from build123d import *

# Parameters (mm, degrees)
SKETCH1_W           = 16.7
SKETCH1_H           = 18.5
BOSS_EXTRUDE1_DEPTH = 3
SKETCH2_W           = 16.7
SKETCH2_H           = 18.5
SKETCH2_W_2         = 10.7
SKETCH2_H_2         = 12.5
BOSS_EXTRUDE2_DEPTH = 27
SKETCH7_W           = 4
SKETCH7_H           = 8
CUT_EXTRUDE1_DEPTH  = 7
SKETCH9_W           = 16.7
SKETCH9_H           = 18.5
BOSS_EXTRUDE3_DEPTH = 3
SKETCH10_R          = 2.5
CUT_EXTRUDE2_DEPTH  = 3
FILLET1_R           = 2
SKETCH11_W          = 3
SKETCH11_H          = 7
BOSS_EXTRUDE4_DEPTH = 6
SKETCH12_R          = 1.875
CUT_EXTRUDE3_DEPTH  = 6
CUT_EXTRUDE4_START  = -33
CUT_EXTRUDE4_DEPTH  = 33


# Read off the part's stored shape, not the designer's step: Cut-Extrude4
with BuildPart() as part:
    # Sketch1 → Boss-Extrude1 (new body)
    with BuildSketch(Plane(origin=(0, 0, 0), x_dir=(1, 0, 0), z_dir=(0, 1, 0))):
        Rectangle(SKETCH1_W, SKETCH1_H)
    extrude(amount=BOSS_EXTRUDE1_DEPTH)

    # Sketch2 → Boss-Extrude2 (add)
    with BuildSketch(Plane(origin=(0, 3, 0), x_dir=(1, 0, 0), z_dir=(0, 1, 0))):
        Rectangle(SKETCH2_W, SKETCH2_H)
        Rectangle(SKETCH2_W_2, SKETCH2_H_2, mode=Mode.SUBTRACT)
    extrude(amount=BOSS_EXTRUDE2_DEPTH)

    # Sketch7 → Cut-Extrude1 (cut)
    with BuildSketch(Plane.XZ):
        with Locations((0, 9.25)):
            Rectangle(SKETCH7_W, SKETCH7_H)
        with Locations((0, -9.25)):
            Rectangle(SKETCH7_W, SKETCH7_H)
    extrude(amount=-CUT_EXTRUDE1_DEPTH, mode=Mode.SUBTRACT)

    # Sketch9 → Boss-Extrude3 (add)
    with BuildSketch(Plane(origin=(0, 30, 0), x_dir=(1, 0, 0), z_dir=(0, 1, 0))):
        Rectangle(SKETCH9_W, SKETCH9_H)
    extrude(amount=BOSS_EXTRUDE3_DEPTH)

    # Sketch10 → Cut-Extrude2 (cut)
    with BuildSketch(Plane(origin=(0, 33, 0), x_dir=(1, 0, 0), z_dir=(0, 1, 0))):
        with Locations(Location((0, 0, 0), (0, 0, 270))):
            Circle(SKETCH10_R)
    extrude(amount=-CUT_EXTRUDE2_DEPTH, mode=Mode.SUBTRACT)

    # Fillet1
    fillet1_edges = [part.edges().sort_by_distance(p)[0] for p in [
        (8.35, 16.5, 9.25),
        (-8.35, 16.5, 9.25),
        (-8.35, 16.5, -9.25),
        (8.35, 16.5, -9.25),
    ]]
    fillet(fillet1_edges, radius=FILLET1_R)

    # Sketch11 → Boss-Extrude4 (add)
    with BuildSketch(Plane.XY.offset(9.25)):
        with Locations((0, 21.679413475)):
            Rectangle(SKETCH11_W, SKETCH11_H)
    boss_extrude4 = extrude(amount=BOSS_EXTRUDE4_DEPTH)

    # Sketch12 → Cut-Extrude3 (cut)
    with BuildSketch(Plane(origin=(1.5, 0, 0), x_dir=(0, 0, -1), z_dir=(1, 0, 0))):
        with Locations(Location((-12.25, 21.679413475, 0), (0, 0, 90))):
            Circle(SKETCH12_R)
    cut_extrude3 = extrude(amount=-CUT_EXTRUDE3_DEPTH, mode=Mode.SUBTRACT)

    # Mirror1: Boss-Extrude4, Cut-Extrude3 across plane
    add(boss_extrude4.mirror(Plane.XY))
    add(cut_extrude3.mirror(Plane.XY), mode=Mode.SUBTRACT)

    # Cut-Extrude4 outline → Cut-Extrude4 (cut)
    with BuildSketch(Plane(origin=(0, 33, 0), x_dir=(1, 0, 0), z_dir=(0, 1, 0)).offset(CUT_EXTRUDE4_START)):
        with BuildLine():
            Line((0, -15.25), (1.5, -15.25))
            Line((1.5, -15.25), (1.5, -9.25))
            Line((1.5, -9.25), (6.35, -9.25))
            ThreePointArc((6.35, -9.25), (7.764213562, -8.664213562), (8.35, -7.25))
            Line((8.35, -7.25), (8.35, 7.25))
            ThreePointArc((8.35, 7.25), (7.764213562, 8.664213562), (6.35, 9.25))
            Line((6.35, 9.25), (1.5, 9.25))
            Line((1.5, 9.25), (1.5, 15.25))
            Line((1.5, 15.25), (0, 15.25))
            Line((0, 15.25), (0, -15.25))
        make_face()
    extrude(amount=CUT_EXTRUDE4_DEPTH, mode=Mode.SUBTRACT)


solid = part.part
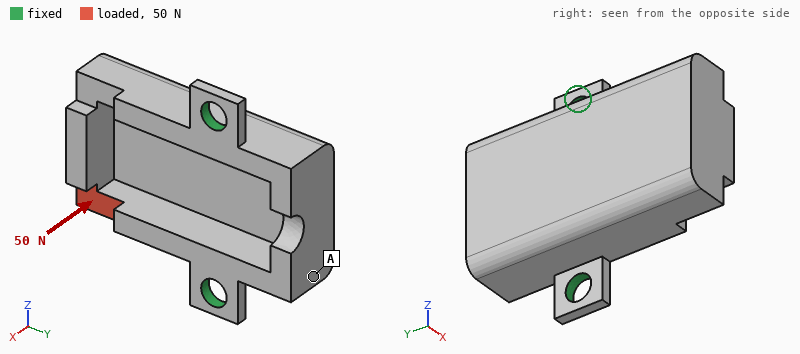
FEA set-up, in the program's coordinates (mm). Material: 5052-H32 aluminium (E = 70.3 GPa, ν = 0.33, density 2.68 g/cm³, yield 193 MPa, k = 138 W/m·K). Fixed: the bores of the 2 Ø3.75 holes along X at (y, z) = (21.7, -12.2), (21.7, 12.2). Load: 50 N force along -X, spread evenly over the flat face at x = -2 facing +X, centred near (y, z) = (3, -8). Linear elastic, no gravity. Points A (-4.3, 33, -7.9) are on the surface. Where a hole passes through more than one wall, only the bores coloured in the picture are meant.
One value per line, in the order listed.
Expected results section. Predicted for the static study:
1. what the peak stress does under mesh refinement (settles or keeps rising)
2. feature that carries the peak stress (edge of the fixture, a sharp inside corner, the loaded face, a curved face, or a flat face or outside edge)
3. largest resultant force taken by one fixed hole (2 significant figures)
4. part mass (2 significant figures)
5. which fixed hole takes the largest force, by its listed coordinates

keeps rising
edge of the fixture
47 N
8.6 g
(21.7, -12.2)
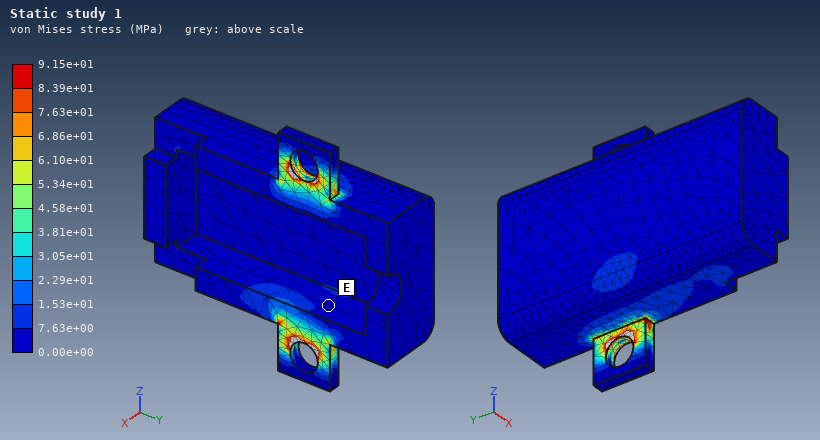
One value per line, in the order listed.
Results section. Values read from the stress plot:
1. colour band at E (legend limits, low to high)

0.00e+00 to 7.63e+00 MPa
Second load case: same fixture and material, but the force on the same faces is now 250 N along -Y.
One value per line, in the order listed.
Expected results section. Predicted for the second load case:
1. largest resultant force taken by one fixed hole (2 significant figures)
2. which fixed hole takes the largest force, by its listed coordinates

220 N
(21.7, -12.2)
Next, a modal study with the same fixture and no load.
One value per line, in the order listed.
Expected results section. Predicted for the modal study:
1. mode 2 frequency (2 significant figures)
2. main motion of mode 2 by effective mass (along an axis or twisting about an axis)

9000 Hz
along Z
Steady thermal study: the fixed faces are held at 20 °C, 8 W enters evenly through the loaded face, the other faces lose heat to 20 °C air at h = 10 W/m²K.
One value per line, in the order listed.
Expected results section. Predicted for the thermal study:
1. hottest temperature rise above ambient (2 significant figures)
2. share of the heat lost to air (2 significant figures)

31 K
3.8 %
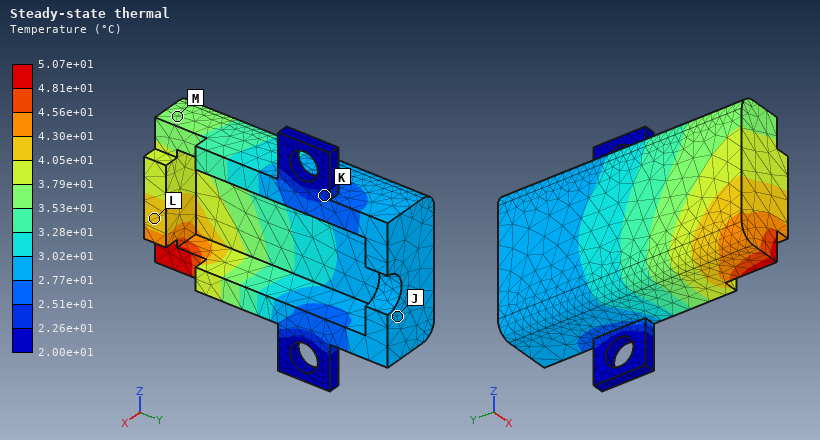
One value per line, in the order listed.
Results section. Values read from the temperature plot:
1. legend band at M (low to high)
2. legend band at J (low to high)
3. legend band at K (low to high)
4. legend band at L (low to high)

3.53e+01 to 3.79e+01 °C
2.77e+01 to 3.02e+01 °C
2.26e+01 to 2.51e+01 °C
4.05e+01 to 4.30e+01 °C
